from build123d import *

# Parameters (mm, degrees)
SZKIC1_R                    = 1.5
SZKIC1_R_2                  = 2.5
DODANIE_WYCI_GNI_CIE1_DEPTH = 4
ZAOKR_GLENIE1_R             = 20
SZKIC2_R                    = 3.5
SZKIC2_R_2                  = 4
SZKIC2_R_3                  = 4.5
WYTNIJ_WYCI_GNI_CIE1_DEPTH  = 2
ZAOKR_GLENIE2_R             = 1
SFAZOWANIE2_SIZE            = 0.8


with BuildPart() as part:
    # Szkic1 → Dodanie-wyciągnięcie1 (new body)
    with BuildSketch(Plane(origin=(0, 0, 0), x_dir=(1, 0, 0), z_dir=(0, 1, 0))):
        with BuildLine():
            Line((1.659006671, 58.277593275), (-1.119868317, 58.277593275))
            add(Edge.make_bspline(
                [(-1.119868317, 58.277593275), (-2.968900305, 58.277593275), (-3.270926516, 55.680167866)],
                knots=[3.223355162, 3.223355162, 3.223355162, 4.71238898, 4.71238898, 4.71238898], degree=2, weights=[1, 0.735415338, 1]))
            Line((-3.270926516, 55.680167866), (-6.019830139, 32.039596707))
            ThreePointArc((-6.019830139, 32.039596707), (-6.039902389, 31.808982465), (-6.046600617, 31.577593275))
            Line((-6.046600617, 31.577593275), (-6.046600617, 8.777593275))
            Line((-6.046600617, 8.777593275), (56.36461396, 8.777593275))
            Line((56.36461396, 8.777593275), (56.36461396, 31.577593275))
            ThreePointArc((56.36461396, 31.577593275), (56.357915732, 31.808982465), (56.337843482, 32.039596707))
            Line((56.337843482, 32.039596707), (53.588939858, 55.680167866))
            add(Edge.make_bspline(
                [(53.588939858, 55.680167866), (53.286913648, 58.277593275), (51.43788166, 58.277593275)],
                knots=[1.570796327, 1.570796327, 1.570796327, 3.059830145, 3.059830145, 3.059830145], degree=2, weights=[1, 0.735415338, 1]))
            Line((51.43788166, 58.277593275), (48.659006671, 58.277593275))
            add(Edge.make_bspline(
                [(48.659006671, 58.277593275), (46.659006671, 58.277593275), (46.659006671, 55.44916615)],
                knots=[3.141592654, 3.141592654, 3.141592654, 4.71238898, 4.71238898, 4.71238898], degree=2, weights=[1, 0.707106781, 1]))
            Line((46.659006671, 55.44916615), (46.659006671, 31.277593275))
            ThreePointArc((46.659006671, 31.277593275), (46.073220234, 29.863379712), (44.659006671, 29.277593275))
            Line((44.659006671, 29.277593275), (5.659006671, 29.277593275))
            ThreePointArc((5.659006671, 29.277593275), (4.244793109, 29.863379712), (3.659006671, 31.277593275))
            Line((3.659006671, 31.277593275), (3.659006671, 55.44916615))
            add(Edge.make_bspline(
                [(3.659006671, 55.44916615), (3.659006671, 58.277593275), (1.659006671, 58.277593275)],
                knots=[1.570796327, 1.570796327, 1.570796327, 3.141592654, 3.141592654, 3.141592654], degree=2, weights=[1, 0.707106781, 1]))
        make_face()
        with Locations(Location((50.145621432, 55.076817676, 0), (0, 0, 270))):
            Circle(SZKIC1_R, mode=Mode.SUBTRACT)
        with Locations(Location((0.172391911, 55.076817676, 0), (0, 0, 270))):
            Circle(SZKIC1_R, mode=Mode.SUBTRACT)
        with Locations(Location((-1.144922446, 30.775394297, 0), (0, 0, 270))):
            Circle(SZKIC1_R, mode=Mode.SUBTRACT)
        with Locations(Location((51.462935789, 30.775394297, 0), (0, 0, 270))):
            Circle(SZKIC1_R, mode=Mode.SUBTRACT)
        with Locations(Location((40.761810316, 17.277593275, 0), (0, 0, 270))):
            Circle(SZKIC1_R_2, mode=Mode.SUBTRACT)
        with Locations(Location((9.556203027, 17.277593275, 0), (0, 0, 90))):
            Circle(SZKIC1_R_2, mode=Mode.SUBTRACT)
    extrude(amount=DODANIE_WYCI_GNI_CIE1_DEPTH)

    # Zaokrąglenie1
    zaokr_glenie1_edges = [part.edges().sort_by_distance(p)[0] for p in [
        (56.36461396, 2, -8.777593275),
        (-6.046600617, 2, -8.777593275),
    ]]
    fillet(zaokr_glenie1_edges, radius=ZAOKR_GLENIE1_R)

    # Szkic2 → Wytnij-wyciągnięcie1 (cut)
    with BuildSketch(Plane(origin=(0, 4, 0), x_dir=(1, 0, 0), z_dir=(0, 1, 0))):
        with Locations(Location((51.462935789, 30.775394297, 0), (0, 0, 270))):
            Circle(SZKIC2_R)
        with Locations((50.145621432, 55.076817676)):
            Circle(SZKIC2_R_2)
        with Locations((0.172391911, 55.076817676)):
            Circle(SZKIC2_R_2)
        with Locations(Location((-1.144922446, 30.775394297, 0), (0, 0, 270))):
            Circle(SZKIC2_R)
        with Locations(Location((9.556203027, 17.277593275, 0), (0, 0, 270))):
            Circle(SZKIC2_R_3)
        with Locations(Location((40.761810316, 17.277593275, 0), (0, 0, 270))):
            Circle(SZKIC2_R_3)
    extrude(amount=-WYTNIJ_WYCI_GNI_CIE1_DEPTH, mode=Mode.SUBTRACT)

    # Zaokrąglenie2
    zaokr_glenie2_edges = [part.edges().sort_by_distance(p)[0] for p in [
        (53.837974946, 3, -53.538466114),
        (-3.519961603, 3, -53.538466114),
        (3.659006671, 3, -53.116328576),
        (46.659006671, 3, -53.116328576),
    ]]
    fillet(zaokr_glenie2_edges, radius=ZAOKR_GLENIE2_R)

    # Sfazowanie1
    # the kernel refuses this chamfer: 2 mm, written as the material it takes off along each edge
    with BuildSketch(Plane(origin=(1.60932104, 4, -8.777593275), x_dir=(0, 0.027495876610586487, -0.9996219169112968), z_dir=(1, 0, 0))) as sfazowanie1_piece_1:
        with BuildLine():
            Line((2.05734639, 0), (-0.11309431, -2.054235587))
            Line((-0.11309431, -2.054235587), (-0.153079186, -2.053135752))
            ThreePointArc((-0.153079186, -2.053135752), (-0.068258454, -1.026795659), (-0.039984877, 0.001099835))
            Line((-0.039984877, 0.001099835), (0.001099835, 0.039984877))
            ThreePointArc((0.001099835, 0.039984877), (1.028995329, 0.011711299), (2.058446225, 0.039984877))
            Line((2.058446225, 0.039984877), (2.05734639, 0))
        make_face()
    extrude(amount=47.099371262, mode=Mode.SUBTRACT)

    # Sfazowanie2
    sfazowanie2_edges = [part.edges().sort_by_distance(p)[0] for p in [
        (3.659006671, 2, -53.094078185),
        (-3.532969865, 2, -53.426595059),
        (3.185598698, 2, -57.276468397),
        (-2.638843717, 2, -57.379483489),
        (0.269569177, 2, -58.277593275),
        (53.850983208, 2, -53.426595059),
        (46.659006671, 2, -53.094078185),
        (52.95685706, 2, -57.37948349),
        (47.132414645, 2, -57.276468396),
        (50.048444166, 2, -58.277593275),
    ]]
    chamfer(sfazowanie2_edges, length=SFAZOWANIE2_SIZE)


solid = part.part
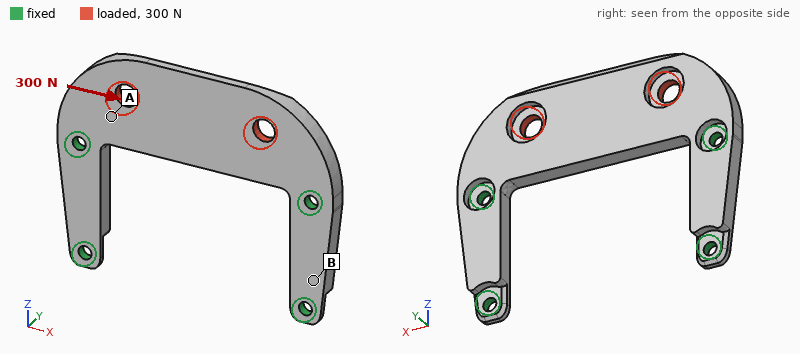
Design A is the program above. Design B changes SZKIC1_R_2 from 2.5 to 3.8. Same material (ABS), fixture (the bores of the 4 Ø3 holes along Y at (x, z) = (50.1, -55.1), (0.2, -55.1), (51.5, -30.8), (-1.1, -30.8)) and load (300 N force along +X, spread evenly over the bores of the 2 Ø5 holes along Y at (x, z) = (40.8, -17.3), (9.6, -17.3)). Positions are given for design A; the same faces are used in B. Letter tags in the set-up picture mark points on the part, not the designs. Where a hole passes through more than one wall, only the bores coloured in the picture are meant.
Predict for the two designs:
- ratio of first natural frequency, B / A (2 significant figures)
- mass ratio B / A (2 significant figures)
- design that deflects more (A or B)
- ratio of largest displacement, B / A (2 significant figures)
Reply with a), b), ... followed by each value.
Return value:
a) 1.0
b) 0.98
c) B
d) 1.1
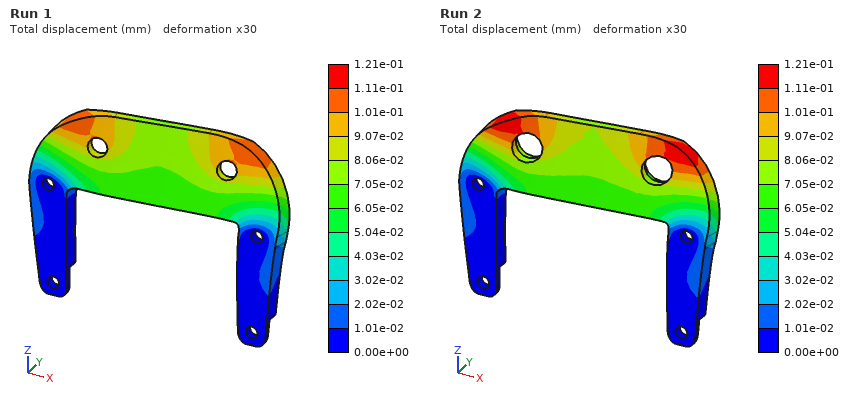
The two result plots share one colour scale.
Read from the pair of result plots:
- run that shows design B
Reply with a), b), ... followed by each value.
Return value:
a) Run 2
